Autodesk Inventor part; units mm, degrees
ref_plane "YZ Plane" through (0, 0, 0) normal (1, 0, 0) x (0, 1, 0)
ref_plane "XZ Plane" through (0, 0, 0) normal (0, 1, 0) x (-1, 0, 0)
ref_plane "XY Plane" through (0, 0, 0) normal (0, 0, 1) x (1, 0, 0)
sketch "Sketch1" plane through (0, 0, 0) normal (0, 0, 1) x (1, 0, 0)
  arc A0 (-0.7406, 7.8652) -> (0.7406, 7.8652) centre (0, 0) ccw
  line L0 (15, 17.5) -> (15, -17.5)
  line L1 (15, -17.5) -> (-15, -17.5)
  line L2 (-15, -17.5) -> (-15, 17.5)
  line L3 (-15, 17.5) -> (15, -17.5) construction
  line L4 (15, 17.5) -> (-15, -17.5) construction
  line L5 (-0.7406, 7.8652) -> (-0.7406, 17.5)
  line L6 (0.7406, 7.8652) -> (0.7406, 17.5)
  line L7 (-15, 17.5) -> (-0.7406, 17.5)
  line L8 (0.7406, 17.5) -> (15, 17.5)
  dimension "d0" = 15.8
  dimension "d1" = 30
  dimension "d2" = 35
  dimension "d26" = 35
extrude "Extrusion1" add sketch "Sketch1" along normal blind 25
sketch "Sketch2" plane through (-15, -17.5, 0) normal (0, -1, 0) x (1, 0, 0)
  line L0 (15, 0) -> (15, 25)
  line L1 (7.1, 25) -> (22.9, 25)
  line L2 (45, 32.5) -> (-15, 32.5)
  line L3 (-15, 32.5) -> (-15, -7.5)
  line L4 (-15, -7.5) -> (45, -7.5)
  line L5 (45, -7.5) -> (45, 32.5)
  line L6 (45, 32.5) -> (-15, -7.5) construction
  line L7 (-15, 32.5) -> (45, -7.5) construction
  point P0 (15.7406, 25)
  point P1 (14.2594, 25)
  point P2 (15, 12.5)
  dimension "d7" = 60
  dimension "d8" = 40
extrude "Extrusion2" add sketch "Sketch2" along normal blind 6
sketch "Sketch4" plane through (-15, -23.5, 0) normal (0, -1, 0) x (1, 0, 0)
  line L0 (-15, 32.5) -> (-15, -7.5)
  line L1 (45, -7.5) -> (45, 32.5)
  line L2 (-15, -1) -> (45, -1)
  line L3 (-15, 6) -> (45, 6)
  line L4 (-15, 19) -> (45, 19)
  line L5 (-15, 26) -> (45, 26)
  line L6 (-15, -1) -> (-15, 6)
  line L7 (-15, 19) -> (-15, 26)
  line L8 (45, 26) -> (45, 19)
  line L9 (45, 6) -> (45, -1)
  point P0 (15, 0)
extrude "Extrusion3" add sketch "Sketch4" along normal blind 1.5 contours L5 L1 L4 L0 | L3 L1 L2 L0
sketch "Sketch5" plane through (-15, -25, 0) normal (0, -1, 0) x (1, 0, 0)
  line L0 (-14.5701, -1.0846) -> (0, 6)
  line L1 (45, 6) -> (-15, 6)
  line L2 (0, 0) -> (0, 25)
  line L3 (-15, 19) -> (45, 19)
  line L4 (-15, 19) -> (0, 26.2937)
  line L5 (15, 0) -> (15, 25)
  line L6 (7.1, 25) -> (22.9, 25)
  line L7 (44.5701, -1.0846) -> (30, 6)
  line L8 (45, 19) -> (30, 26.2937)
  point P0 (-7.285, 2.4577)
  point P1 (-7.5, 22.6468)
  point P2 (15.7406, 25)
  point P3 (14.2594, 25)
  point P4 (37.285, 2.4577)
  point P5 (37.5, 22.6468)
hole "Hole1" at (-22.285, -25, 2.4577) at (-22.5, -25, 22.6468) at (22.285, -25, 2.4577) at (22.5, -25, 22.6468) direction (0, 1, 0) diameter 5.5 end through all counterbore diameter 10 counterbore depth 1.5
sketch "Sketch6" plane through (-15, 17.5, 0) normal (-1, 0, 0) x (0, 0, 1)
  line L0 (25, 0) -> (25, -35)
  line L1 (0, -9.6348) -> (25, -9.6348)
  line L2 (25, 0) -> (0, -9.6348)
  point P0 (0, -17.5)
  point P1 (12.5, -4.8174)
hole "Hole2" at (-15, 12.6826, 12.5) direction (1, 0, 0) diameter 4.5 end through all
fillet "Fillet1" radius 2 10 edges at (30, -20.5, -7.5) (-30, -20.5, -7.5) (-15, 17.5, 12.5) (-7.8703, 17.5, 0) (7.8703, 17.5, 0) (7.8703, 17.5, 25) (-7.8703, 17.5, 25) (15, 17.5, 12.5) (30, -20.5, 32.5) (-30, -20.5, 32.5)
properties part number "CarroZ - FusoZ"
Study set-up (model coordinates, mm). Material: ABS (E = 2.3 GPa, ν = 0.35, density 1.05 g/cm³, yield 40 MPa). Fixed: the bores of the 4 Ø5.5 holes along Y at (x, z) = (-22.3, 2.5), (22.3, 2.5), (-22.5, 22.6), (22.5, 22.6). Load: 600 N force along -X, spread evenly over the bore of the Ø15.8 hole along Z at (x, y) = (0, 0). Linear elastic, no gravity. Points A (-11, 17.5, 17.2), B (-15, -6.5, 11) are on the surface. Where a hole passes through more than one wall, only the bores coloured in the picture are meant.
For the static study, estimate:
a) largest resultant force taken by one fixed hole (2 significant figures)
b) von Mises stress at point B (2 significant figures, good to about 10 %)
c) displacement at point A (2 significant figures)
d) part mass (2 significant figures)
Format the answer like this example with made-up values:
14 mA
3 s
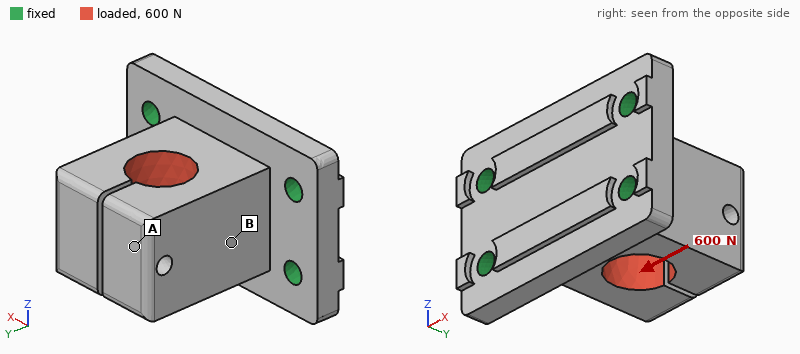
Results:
230 N
4.1 MPa
0.27 mm
37 g
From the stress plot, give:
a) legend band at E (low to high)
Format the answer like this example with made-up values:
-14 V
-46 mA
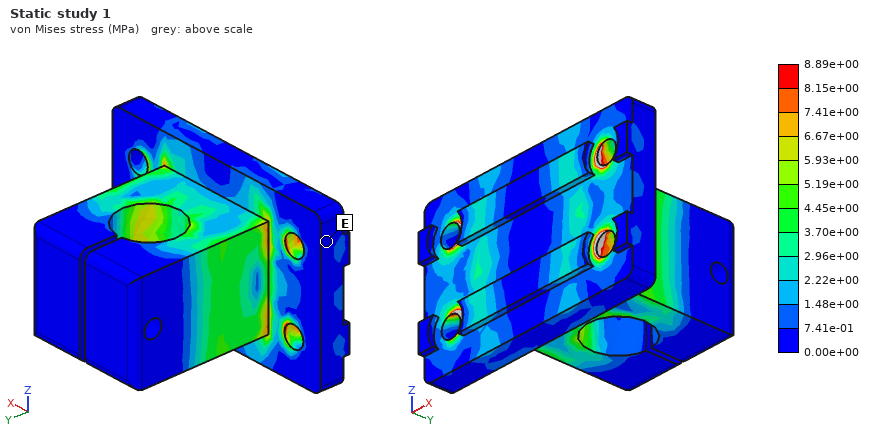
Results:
0.00e+00 to 7.41e-01 MPa
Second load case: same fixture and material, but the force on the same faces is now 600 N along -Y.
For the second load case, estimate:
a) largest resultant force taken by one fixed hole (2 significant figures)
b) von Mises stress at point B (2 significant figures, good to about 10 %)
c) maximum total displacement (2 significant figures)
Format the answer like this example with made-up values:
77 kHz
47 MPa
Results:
170 N
1.7 MPa
0.18 mm
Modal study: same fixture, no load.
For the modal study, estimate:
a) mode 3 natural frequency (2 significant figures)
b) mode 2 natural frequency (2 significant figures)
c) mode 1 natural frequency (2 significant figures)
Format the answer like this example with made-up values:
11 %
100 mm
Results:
1800 Hz
1700 Hz
1700 Hz
